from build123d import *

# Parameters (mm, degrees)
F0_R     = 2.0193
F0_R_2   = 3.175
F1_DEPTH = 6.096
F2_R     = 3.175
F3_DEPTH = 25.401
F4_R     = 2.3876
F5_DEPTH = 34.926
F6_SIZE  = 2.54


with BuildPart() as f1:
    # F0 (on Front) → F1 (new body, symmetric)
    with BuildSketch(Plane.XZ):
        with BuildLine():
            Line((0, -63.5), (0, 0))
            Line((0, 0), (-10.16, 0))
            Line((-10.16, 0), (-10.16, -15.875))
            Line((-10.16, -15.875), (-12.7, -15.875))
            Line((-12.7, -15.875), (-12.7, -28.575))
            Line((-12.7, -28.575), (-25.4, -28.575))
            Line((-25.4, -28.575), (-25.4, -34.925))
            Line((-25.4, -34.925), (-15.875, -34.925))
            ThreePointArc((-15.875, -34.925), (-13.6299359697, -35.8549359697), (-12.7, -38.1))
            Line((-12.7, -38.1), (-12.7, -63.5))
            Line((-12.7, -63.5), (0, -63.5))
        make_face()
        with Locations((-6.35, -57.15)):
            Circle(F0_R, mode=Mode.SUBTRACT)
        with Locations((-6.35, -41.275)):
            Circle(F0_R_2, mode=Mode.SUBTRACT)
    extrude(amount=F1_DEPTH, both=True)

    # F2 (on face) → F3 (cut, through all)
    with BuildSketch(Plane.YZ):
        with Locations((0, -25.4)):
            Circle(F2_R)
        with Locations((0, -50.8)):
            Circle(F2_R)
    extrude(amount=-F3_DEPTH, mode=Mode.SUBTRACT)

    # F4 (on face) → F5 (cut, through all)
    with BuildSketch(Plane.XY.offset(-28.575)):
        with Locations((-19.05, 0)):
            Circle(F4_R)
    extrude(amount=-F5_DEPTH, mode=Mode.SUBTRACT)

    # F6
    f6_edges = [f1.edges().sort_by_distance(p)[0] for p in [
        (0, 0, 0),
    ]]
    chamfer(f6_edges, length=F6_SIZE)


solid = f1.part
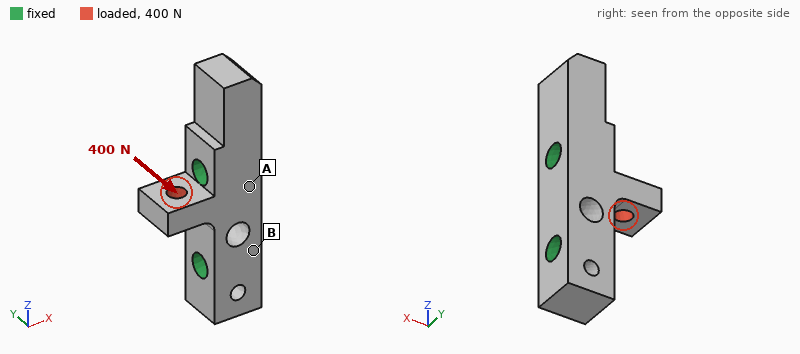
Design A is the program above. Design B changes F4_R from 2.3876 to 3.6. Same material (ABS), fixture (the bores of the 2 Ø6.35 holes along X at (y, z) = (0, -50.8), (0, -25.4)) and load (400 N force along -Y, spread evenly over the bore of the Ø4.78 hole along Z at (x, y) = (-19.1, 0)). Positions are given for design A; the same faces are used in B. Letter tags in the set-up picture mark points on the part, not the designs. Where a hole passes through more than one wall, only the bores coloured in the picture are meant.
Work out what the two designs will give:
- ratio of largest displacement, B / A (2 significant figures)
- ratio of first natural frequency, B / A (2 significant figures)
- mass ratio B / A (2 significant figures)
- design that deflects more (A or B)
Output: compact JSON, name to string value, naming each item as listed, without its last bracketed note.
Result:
{"ratio of largest displacement, B / A": "1.4", "ratio of first natural frequency, B / A": "1.00", "mass ratio B / A": "0.98", "design that deflects more": "B"}
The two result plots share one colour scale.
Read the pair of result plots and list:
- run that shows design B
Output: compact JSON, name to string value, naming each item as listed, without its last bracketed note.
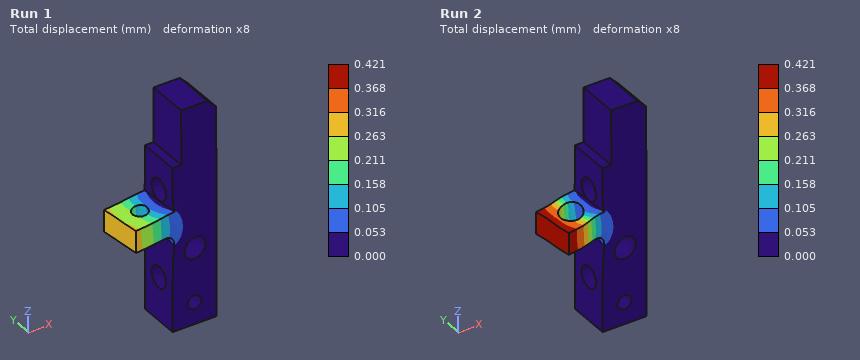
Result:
{"run that shows design B": "Run 2"}
